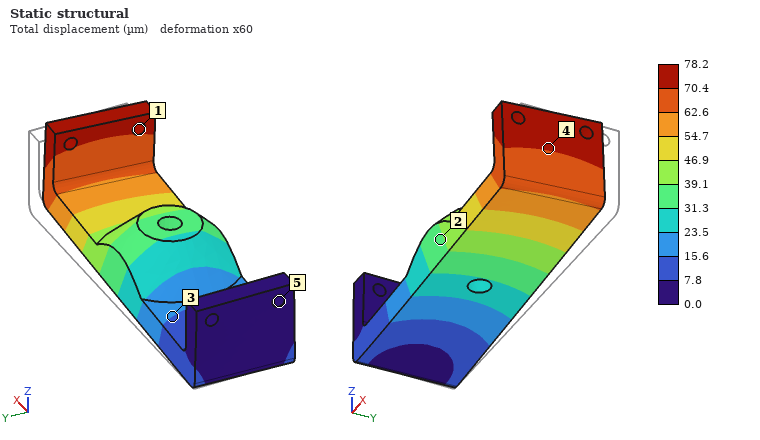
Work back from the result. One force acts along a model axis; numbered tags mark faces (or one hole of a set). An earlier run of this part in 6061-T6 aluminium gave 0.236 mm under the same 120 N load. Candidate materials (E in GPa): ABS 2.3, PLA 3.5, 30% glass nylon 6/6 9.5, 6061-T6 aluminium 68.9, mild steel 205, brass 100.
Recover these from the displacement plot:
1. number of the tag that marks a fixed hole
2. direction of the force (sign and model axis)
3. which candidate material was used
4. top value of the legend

5
-Y
mild steel
78.2 µm
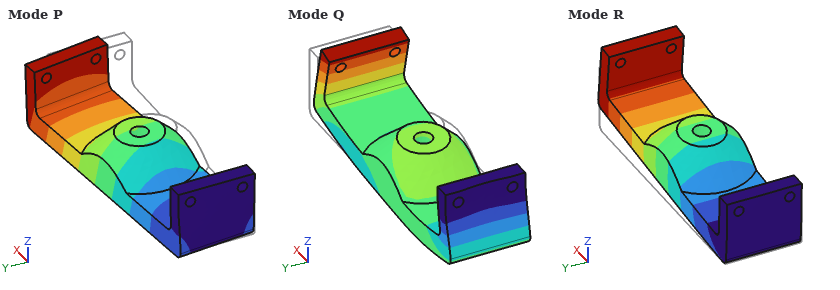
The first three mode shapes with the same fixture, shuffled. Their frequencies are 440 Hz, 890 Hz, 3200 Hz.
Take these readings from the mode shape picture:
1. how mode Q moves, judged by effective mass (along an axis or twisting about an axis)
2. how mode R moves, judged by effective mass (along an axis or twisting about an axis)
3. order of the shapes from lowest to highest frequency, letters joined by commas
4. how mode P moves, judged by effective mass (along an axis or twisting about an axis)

along X
along Z
R, P, Q
along Y
